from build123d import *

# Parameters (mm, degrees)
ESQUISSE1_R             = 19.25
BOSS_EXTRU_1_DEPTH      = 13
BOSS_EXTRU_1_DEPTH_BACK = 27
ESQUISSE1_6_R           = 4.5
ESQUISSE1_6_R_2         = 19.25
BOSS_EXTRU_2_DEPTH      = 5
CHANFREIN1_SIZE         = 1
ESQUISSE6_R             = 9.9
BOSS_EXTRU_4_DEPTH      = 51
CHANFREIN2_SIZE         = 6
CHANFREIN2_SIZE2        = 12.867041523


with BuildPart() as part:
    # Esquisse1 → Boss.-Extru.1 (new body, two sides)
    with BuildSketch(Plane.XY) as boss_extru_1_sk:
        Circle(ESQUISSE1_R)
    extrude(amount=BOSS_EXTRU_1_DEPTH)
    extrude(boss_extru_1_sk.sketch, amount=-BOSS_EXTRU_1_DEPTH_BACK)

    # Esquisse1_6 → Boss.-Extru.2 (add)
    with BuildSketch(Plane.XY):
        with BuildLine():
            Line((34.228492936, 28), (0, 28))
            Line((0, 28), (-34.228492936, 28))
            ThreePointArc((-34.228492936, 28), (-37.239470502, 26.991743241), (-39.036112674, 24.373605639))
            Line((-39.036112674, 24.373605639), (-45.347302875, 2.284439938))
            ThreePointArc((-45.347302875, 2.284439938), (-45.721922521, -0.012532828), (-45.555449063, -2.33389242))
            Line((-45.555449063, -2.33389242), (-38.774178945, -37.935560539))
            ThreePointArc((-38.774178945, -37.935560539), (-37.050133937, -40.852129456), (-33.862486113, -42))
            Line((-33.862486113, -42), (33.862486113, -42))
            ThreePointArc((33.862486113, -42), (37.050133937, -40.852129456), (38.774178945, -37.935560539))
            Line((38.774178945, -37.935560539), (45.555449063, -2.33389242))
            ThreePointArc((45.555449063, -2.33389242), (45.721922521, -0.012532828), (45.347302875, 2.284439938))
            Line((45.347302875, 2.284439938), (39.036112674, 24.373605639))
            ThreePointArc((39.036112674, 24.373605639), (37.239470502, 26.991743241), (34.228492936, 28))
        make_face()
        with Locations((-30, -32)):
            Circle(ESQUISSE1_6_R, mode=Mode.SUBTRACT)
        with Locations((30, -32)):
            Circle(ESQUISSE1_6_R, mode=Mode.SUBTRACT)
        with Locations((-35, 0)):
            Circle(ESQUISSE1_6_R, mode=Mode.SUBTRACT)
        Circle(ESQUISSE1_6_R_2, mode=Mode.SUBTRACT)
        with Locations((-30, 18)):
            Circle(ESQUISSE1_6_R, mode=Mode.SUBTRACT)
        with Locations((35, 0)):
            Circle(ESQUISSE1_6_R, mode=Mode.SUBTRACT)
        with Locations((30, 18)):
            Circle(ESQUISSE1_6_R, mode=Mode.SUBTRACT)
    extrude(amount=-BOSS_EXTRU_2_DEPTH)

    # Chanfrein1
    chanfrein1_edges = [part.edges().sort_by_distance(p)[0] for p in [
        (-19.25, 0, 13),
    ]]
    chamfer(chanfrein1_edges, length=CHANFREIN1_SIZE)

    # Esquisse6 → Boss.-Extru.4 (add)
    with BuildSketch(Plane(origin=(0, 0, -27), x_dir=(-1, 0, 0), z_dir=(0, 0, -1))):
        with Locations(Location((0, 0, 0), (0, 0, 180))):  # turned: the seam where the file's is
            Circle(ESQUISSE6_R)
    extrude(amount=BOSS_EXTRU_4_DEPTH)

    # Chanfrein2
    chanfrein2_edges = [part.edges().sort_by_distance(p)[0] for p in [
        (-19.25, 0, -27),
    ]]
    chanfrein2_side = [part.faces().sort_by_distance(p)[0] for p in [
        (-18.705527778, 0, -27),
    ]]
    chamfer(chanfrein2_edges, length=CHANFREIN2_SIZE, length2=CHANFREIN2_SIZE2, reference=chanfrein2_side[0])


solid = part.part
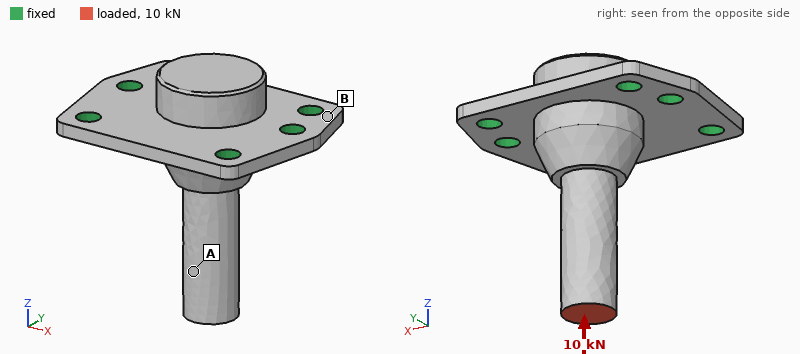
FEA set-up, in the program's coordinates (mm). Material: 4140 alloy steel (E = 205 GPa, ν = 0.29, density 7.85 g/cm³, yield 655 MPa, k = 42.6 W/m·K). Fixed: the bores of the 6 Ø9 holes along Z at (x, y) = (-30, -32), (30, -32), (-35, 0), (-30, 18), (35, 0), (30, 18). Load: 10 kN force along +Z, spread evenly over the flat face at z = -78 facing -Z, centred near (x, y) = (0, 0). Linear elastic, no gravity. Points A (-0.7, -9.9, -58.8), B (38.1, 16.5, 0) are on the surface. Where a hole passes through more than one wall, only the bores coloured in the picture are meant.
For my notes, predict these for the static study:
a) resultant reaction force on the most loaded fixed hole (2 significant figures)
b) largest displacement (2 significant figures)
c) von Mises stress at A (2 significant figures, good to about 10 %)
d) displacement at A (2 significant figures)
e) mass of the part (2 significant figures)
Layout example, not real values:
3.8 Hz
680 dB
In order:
2.2 kN
32 µm
32 MPa
28 µm
630 g
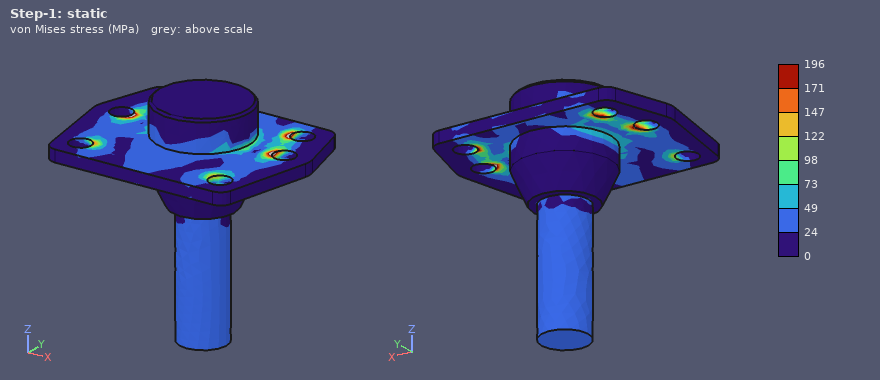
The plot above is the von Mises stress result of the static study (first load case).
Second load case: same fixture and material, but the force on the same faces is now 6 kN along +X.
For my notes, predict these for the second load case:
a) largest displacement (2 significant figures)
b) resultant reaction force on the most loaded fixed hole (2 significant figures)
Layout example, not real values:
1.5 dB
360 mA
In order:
0.37 mm
4.8 kN
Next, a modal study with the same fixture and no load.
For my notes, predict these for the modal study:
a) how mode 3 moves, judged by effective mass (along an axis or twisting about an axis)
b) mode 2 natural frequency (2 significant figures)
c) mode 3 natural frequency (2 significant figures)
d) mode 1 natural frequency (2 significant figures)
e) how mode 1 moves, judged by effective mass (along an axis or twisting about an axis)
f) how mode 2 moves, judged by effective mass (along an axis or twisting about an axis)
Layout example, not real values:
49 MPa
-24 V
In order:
along Z
3100 Hz
5300 Hz
2300 Hz
along Y
along X
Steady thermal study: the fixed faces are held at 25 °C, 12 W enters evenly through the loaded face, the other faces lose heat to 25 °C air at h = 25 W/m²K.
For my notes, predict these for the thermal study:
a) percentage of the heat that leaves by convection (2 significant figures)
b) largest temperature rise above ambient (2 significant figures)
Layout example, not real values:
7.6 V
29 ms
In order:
33 %
53 K
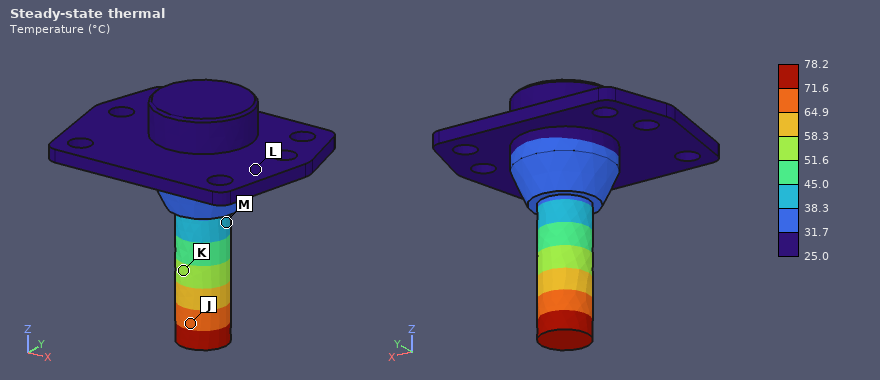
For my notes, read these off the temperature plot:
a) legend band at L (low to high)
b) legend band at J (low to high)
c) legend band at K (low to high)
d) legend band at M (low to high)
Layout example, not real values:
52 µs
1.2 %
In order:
25.0 to 31.7 °C
64.9 to 71.6 °C
51.6 to 58.3 °C
38.3 to 45.0 °C
